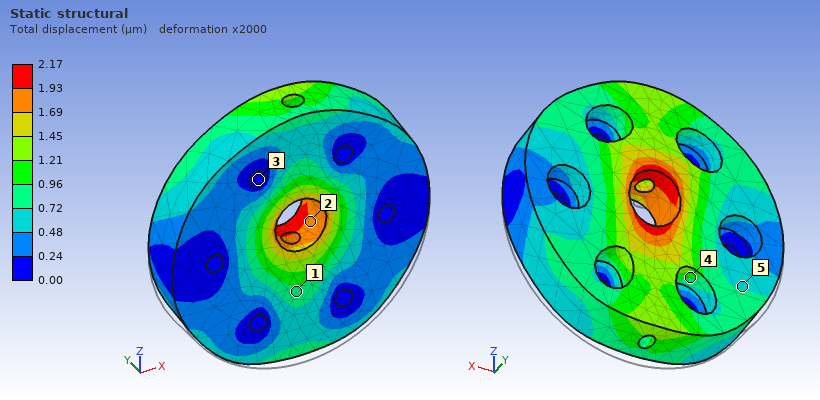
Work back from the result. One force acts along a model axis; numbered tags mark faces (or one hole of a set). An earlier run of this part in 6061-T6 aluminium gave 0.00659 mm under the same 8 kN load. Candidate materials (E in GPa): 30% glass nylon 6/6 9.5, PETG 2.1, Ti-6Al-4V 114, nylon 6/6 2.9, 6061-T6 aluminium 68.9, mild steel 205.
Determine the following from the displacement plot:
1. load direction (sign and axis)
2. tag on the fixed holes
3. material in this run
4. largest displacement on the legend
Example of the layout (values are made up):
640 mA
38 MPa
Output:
+Z
3
mild steel
2.17 µm
